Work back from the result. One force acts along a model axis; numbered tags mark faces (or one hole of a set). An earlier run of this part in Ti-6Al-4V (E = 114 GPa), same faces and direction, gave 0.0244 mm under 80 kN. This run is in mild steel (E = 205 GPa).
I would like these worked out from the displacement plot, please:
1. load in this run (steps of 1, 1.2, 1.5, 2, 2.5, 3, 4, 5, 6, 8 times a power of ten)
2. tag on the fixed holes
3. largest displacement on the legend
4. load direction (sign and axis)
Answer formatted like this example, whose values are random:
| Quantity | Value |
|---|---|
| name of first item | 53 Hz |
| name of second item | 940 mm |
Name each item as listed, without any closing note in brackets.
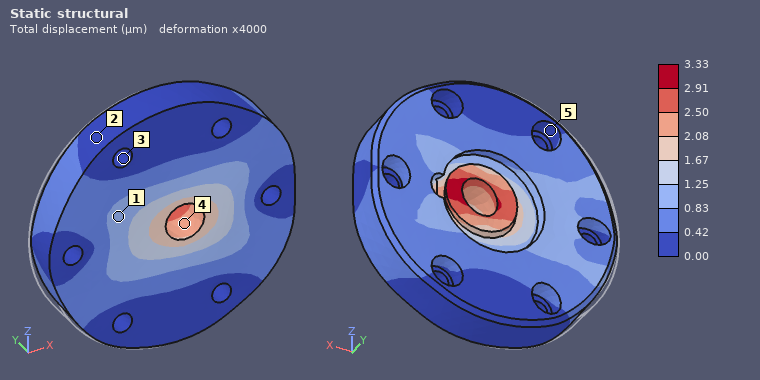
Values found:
| Quantity | Value |
|---|---|
| load in this run | 20 kN |
| tag on the fixed holes | 3 |
| largest displacement on the legend | 3.33 µm |
| load direction | +X |
